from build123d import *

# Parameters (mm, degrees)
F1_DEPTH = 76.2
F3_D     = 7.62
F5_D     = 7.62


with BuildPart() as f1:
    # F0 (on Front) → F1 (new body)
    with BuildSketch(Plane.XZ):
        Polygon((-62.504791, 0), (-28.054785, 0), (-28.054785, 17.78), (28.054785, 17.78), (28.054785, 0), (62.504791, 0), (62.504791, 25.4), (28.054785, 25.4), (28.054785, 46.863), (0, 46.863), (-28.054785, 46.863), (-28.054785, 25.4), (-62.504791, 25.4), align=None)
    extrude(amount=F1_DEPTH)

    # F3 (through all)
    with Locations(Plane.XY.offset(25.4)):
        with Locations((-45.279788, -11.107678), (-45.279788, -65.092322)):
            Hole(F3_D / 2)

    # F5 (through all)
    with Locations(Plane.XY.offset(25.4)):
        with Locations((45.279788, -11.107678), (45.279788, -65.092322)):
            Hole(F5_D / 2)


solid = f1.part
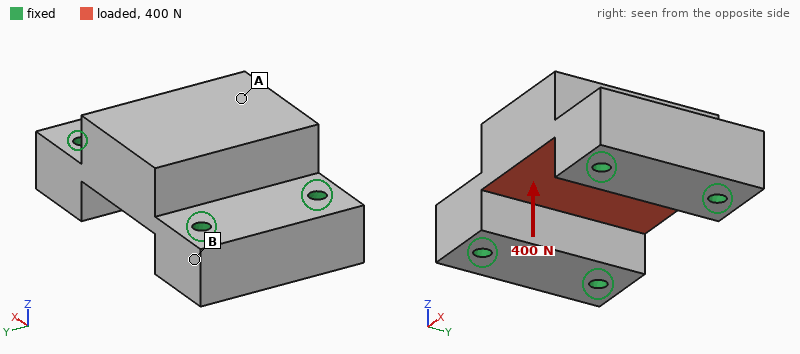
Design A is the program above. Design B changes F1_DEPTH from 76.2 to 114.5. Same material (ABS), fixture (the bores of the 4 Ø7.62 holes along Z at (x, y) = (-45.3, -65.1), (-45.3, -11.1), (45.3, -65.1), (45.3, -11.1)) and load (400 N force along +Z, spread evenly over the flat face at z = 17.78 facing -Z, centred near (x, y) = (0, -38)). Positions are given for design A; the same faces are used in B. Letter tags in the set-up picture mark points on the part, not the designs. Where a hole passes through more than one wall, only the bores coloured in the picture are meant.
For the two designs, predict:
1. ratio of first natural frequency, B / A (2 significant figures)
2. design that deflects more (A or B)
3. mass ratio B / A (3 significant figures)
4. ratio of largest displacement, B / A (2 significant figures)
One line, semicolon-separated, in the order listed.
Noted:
0.63; B; 1.51; 1.8
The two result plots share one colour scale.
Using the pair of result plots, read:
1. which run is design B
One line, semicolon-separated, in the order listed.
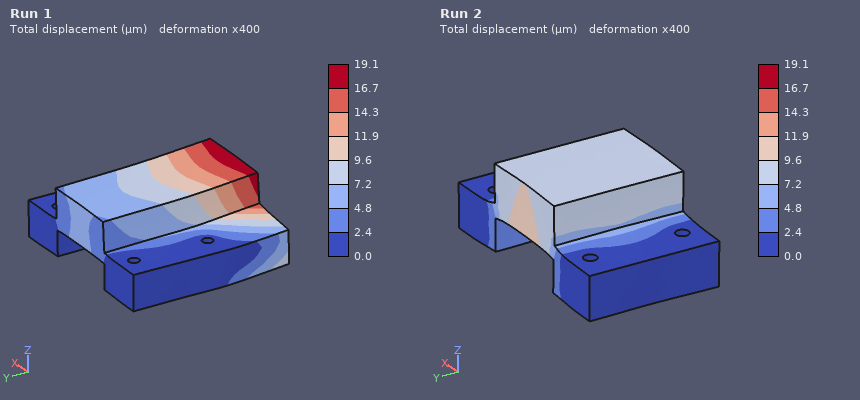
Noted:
Run 1
